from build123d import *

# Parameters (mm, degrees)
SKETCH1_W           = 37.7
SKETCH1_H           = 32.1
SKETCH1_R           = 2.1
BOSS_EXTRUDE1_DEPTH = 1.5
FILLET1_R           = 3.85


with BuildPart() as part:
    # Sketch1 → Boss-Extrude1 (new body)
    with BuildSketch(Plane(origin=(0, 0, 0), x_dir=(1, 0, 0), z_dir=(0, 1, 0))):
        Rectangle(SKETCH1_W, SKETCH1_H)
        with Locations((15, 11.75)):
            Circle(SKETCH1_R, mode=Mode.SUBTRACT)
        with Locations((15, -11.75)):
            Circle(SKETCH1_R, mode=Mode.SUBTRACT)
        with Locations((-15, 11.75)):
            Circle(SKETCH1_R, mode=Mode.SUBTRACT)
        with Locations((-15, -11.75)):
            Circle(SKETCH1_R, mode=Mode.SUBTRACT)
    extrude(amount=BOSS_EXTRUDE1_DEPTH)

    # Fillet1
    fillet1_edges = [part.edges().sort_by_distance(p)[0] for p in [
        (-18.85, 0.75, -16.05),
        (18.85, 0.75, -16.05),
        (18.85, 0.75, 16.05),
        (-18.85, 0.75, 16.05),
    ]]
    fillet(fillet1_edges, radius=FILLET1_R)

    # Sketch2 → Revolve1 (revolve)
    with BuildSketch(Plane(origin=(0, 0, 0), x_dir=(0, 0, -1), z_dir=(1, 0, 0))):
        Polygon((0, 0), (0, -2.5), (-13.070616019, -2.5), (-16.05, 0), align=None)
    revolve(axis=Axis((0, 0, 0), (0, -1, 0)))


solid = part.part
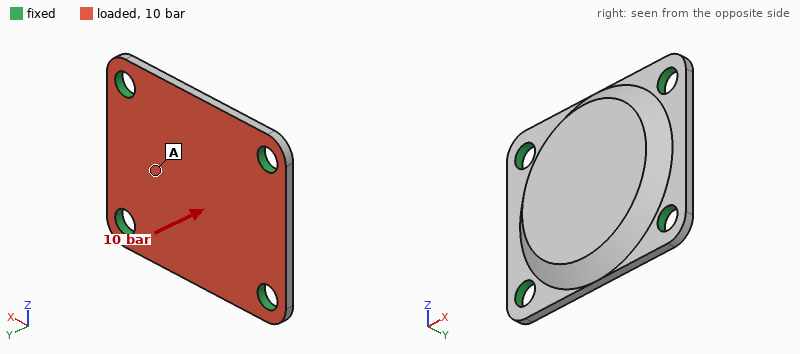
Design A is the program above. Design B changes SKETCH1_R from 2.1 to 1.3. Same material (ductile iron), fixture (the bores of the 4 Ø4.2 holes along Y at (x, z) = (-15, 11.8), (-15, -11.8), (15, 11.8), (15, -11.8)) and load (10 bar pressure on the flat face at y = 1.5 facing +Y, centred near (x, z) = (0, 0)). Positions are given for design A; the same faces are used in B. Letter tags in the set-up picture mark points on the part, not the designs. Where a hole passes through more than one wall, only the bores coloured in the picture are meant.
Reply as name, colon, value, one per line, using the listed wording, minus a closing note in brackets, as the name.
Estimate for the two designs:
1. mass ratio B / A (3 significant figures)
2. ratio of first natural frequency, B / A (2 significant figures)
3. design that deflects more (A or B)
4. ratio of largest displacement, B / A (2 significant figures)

mass ratio B / A: 1.02
ratio of first natural frequency, B / A: 0.84
design that deflects more: B
ratio of largest displacement, B / A: 1.4
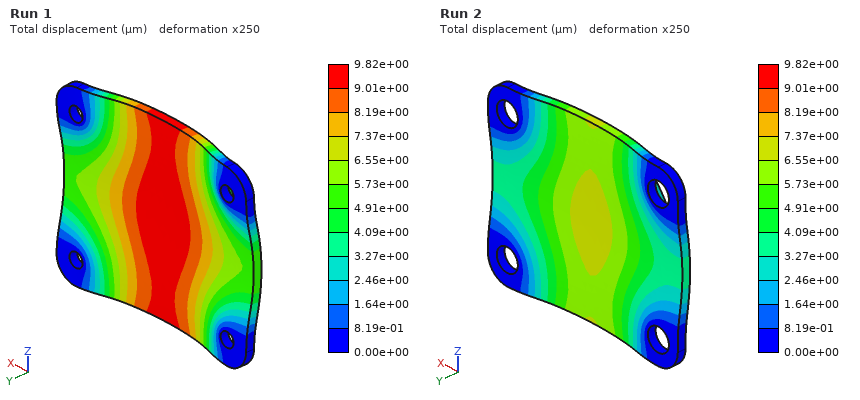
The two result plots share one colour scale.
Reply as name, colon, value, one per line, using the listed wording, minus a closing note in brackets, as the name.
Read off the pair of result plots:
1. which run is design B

which run is design B: Run 1
